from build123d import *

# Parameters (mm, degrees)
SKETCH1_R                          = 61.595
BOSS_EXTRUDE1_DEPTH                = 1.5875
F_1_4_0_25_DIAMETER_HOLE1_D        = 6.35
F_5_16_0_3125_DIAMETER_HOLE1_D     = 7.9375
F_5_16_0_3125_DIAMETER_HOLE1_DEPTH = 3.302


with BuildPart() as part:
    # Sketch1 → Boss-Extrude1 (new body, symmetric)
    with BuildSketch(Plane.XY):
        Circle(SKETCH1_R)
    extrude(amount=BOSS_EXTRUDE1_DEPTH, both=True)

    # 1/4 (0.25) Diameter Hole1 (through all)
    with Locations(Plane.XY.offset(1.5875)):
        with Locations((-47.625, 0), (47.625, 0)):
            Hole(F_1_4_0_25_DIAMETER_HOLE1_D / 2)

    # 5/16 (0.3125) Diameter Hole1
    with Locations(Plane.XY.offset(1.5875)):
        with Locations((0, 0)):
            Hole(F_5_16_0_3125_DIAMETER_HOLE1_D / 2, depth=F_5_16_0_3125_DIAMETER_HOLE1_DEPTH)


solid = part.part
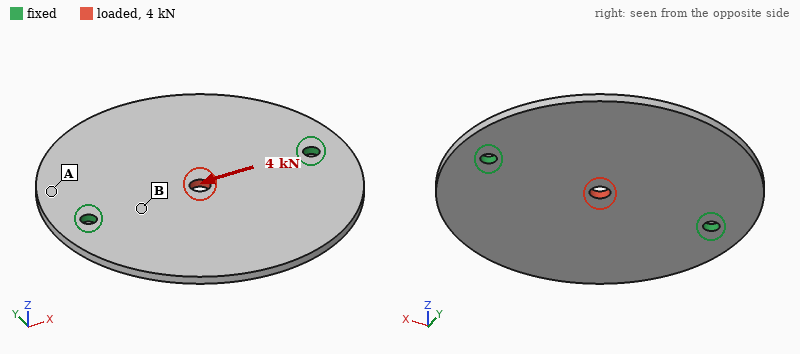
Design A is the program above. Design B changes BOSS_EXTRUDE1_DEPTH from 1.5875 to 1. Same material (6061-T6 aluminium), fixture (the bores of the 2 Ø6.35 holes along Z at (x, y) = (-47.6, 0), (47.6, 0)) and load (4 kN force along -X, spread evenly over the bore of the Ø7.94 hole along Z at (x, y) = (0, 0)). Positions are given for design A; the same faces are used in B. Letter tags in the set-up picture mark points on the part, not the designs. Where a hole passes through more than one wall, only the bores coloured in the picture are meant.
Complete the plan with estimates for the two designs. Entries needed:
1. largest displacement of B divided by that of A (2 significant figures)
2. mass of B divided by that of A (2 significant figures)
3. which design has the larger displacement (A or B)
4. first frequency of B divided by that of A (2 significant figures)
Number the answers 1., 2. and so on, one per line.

1. 1.6
2. 0.63
3. B
4. 0.64
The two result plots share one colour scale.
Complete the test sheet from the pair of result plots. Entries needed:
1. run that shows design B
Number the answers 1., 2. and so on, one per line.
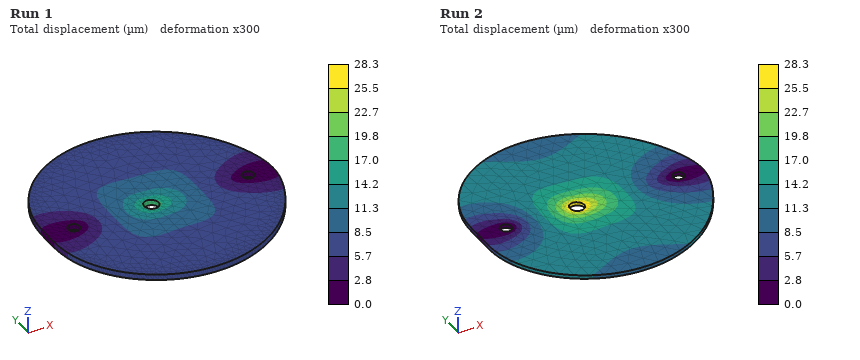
1. Run 2
